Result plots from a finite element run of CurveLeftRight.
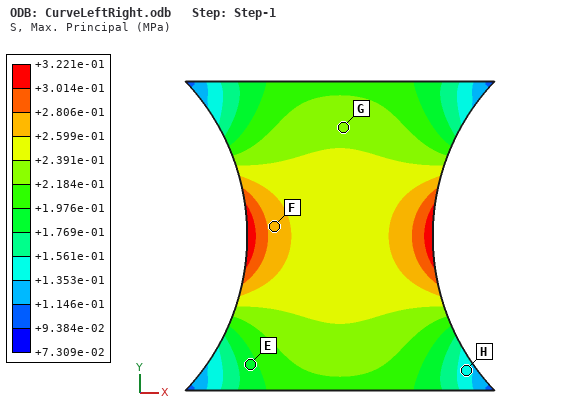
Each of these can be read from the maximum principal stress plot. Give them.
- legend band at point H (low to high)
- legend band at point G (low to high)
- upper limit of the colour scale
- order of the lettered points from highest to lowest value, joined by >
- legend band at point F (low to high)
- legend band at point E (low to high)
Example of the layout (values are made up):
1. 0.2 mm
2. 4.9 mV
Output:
1. +1.353e-01 to +1.561e-01 MPa
2. +2.184e-01 to +2.391e-01 MPa
3. +3.221e-01 MPa
4. F > G > E > H
5. +2.599e-01 to +2.806e-01 MPa
6. +1.769e-01 to +1.976e-01 MPa
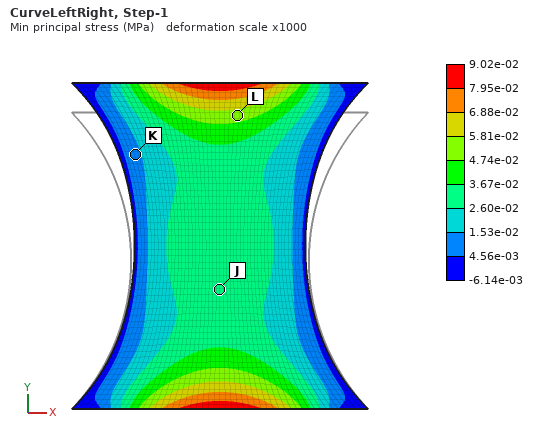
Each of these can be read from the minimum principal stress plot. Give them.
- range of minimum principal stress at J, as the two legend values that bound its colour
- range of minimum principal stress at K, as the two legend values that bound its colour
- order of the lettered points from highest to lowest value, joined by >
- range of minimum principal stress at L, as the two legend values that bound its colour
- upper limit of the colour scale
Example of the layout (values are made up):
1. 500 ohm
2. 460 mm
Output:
1. 2.60e-02 to 3.67e-02 MPa
2. 4.56e-03 to 1.53e-02 MPa
3. L > J > K
4. 4.74e-02 to 5.81e-02 MPa
5. 9.02e-02 MPa
